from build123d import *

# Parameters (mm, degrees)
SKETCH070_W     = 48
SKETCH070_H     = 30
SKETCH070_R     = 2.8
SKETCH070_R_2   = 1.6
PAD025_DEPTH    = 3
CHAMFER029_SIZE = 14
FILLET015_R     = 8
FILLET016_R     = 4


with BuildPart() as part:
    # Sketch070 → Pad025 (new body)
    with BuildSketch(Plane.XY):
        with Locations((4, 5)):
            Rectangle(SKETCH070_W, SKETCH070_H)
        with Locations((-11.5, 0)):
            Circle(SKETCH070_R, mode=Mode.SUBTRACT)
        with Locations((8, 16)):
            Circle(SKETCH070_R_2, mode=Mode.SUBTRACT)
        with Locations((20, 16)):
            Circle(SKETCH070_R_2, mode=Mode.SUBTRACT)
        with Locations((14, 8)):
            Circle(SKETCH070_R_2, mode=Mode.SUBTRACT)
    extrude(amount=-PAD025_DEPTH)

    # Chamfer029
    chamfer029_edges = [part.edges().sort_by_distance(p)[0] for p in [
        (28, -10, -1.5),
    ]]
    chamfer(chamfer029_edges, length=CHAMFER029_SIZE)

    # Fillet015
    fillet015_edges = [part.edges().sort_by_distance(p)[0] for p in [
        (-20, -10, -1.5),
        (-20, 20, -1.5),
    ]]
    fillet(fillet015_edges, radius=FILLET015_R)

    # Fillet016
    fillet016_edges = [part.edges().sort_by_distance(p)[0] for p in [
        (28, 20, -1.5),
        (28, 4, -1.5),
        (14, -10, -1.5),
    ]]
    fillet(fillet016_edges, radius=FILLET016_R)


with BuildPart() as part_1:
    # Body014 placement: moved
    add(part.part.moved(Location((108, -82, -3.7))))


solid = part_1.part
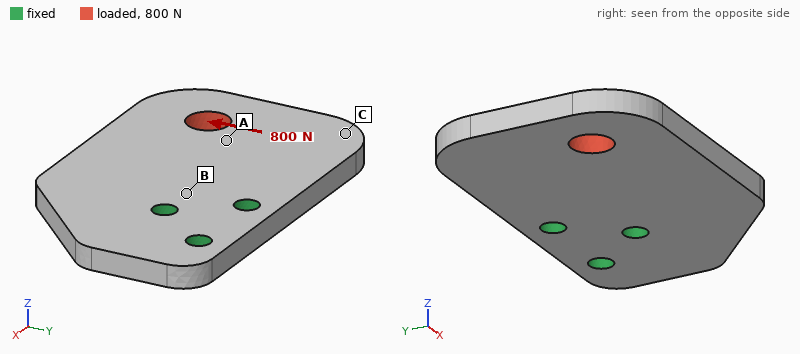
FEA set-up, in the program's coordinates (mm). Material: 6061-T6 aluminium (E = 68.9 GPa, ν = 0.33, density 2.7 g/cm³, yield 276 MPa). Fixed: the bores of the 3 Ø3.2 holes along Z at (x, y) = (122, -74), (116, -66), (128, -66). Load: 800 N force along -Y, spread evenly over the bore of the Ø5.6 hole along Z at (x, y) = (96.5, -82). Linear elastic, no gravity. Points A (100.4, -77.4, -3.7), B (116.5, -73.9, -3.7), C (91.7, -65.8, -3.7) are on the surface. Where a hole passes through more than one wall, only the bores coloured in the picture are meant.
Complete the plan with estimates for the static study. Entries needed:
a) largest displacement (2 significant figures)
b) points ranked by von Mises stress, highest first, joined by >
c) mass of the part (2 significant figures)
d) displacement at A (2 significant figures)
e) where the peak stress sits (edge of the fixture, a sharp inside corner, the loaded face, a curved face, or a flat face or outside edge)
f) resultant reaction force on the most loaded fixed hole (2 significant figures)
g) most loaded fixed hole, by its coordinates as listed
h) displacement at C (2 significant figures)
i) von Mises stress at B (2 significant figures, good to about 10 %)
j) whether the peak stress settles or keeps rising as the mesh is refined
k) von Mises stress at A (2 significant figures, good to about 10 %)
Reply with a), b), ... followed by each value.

a) 41 µm
b) B > A > C
c) 10 g
d) 24 µm
e) edge of the fixture
f) 1.4 kN
g) (116, -66)
h) 34 µm
i) 36 MPa
j) keeps rising
k) 22 MPa
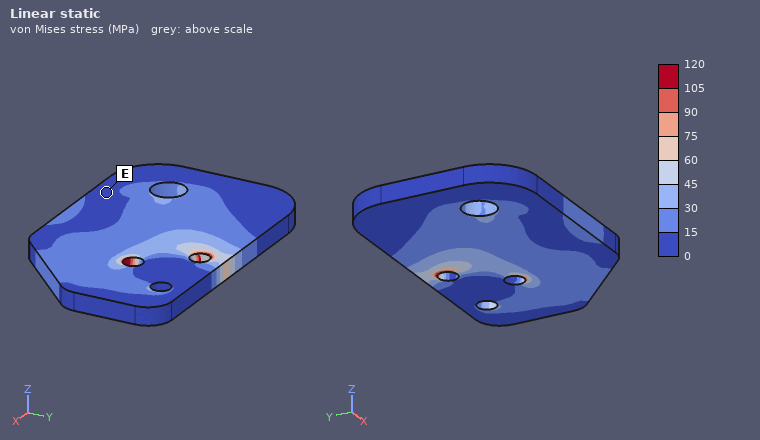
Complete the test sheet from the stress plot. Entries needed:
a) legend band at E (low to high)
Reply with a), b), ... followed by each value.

a) 0 to 15 MPa
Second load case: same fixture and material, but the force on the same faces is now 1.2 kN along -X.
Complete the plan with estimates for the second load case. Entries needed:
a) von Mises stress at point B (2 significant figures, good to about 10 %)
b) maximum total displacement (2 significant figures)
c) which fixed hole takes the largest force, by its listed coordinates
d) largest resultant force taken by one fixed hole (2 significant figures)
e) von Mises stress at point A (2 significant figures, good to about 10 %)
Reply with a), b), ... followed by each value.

a) 41 MPa
b) 31 µm
c) (122, -74)
d) 1.4 kN
e) 25 MPa
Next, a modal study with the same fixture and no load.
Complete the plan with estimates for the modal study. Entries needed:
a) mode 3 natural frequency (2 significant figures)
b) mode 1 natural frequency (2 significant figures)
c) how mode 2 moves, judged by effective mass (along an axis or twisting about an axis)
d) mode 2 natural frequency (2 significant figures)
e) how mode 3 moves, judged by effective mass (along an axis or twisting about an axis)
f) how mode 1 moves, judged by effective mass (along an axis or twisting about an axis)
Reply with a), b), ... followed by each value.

a) 11 kHz
b) 2500 Hz
c) twisting about X
d) 5600 Hz
e) along Z
f) along Z
